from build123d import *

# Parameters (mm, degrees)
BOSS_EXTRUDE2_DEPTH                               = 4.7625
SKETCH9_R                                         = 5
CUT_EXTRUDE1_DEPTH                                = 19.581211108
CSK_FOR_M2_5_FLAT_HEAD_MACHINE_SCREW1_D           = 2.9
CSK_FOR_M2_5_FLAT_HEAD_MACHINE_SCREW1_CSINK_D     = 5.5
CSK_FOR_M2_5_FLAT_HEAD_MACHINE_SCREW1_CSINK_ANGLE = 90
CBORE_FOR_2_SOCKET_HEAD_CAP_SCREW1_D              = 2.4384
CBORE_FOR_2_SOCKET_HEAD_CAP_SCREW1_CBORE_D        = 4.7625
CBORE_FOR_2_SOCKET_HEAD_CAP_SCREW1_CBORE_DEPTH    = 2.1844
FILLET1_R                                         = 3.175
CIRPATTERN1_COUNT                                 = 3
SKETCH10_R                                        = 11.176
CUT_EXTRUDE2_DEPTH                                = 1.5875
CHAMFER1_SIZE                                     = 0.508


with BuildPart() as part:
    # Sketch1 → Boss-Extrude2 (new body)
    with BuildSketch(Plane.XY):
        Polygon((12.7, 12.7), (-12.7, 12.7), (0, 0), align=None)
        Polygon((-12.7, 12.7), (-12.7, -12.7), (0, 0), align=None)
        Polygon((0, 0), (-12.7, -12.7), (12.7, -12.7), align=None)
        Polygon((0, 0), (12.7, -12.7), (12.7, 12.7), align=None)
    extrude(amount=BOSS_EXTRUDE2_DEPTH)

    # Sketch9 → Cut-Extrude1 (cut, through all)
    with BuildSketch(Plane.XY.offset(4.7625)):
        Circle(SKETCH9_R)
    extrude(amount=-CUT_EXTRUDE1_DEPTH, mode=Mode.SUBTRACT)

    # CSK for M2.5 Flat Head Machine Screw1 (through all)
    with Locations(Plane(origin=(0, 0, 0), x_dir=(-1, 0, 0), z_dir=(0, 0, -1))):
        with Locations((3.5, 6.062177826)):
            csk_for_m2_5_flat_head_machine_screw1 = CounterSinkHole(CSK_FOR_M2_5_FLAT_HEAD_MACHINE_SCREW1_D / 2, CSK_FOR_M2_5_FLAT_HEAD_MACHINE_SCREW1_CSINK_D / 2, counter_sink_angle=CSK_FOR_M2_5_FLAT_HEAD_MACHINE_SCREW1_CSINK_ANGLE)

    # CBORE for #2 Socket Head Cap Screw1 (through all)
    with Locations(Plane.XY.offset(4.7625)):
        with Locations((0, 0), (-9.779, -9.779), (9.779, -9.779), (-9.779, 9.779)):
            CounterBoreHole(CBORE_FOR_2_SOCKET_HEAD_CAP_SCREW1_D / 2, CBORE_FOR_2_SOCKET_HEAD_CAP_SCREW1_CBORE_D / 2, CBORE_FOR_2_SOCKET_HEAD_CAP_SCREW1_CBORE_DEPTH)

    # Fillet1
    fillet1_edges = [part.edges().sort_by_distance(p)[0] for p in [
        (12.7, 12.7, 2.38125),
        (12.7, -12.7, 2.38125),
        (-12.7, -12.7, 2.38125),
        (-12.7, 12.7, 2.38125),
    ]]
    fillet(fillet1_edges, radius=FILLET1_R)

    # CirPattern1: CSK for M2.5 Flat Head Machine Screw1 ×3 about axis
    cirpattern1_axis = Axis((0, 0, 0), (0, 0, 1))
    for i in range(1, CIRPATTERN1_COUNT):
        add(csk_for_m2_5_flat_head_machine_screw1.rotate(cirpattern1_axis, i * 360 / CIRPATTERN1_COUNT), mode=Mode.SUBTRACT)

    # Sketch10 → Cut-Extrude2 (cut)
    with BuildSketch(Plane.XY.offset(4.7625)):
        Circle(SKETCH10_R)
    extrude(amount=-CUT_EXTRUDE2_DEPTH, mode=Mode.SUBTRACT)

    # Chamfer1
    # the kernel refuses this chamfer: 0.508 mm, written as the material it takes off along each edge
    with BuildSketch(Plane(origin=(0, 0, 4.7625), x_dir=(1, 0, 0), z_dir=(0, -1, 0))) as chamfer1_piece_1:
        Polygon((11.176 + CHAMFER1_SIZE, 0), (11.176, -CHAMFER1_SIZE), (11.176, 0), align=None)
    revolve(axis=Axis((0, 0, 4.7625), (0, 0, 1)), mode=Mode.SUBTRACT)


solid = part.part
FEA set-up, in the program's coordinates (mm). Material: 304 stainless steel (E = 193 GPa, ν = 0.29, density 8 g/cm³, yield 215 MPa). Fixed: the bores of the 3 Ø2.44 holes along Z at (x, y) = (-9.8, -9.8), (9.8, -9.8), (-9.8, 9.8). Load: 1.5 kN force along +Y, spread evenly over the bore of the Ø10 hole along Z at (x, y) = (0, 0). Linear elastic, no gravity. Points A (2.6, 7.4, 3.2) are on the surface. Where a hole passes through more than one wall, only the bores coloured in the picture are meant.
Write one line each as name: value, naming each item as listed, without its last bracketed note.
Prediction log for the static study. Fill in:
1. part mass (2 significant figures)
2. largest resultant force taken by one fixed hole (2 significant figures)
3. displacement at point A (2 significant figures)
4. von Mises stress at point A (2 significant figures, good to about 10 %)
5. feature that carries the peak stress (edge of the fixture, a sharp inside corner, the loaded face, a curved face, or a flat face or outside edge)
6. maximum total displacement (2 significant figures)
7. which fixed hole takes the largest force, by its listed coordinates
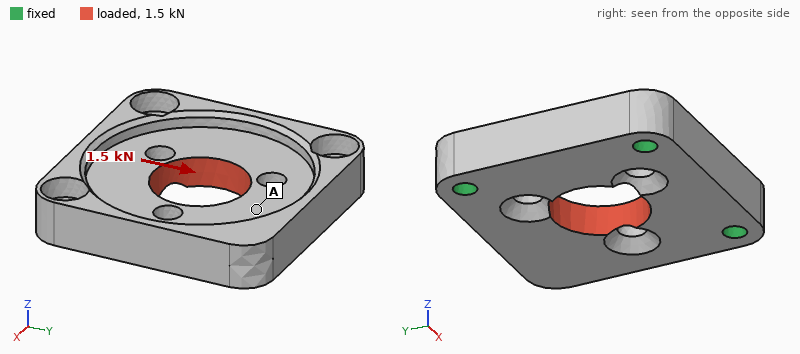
part mass: 15 g
largest resultant force taken by one fixed hole: 660 N
displacement at point A: 2.4 µm
von Mises stress at point A: 10 MPa
feature that carries the peak stress: a curved face
maximum total displacement: 3.3 µm
which fixed hole takes the largest force, by its listed coordinates: (9.8, -9.8)
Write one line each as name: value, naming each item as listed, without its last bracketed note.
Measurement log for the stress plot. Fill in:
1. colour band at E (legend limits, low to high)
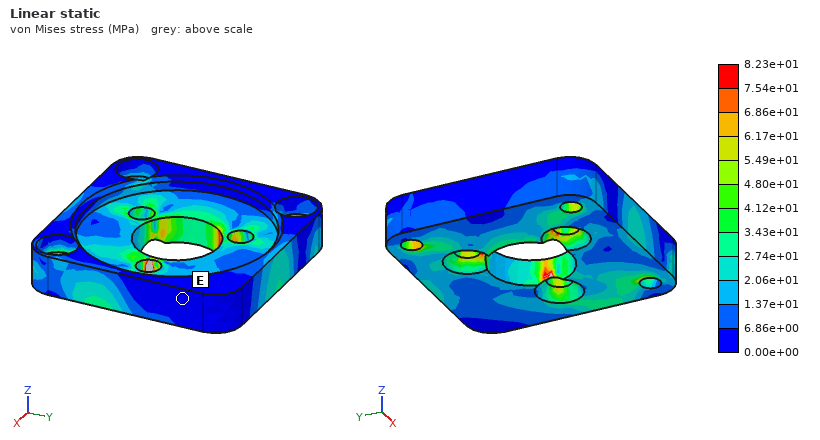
colour band at E: 0.00e+00 to 6.86e+00 MPa
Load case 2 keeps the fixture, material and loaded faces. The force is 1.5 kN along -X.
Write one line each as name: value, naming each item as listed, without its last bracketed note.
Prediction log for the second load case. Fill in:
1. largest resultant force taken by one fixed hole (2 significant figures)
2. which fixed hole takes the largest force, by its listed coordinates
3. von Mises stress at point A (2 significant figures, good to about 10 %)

largest resultant force taken by one fixed hole: 670 N
which fixed hole takes the largest force, by its listed coordinates: (-9.8, 9.8)
von Mises stress at point A: 16 MPa
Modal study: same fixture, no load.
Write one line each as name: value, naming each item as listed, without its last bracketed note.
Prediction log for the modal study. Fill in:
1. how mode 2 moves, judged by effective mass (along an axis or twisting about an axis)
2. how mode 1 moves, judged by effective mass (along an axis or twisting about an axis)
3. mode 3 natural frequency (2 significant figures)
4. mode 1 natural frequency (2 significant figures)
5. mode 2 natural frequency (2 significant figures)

how mode 2 moves, judged by effective mass: along Z
how mode 1 moves, judged by effective mass: along Z
mode 3 natural frequency: 29 kHz
mode 1 natural frequency: 8000 Hz
mode 2 natural frequency: 28 kHz
